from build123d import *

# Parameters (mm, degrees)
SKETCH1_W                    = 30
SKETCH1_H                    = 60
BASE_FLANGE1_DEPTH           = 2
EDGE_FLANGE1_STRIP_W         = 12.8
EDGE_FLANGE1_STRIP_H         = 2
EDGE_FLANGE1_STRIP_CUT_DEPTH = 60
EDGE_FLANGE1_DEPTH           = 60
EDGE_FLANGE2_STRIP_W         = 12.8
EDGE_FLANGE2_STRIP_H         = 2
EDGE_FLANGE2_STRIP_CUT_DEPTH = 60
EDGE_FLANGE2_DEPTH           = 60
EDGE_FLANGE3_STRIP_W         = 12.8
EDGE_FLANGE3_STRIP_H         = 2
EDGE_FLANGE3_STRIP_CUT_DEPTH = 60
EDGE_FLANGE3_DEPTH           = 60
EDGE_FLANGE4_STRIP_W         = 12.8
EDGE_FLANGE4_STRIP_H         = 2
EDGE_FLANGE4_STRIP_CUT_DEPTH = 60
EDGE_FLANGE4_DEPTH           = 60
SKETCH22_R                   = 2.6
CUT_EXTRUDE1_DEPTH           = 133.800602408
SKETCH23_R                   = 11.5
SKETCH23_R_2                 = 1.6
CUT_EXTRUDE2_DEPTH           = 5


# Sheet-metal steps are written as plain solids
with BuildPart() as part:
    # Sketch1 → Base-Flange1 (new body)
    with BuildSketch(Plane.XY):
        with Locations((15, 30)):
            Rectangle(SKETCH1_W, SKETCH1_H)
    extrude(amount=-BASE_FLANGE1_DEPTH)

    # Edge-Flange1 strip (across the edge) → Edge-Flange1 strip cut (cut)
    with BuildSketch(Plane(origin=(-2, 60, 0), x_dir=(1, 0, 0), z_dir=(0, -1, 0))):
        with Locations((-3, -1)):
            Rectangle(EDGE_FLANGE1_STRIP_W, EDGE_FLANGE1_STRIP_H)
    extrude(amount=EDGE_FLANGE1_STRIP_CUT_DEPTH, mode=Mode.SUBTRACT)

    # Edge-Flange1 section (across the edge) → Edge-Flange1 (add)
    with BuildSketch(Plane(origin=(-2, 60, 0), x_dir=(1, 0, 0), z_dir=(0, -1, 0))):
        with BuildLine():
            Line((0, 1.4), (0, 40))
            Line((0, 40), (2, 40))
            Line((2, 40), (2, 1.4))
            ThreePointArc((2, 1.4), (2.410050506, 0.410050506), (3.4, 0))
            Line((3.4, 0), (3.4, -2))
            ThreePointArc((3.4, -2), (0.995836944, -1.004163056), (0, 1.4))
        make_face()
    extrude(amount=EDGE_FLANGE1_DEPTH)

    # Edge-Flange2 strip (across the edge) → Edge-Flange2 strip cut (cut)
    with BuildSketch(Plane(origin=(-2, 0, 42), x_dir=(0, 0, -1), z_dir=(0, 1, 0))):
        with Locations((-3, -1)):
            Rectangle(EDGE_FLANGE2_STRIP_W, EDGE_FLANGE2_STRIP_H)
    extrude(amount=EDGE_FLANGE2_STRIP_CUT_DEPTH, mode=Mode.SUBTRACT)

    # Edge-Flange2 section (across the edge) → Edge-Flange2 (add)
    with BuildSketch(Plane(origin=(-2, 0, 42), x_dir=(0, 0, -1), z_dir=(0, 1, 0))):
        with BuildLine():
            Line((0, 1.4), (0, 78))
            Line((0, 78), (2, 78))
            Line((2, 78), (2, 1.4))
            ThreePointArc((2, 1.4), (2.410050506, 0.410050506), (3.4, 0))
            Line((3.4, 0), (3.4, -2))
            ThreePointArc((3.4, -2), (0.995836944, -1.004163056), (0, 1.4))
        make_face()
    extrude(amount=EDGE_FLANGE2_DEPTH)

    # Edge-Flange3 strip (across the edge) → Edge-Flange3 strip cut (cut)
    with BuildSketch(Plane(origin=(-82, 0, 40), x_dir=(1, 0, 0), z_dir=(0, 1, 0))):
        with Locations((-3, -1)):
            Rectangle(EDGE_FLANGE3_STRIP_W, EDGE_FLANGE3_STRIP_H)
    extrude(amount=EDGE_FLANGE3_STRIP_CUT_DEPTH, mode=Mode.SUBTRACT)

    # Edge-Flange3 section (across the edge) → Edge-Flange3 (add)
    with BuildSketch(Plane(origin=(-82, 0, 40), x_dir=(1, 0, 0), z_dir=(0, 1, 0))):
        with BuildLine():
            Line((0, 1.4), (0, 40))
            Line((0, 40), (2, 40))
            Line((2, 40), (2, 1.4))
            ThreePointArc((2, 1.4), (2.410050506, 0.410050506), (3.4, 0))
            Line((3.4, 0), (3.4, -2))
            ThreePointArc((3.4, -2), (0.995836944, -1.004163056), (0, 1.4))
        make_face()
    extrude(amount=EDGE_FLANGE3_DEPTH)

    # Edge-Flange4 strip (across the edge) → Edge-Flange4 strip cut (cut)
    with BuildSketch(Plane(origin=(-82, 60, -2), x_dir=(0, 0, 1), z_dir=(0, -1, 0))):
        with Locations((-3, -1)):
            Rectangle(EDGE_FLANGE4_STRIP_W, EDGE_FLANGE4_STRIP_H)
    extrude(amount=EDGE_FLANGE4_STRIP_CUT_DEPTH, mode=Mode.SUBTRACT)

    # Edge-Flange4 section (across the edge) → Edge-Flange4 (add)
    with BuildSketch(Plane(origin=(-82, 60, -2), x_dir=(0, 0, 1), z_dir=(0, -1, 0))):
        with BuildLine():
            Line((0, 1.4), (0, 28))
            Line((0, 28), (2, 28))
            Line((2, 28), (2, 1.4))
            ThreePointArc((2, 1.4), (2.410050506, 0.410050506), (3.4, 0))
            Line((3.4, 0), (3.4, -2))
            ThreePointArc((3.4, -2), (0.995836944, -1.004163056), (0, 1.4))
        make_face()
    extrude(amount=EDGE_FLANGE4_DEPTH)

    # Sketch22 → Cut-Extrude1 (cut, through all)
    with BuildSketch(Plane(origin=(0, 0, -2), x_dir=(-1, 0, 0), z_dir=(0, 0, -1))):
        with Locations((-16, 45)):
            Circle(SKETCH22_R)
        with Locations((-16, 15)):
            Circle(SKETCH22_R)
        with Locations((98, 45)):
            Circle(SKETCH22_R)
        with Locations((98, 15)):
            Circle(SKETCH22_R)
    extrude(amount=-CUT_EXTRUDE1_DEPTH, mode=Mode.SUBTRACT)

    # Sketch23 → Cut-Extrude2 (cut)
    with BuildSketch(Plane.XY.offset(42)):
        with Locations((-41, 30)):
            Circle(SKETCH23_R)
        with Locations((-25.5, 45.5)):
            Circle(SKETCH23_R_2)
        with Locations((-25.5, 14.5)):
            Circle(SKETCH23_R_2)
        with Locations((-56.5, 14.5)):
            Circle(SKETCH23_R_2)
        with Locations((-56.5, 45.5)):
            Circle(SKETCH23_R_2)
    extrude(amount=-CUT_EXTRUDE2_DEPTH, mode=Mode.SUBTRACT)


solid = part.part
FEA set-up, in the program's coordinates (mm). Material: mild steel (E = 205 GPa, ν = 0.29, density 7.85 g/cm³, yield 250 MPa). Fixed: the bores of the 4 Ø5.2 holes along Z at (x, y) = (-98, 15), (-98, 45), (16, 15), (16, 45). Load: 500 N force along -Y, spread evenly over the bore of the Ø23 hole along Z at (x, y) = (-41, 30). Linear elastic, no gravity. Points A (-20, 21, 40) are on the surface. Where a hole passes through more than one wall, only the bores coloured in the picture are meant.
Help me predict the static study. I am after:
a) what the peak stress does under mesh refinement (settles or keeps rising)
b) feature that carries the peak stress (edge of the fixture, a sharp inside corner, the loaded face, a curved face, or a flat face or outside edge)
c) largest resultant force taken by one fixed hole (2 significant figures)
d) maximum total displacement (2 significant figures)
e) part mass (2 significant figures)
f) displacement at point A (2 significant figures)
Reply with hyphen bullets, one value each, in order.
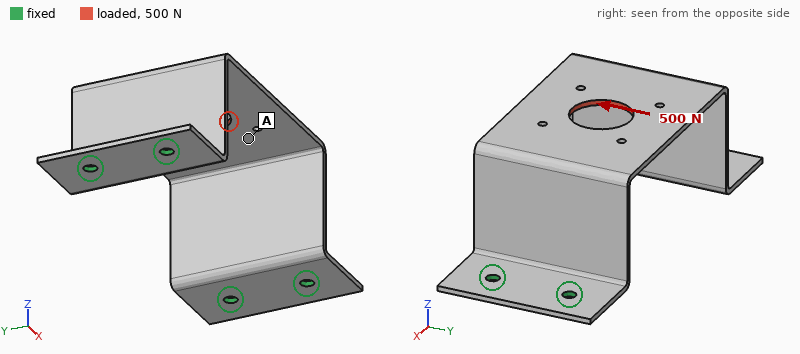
- keeps rising
- edge of the fixture
- 350 N
- 0.16 mm
- 200 g
- 0.13 mm
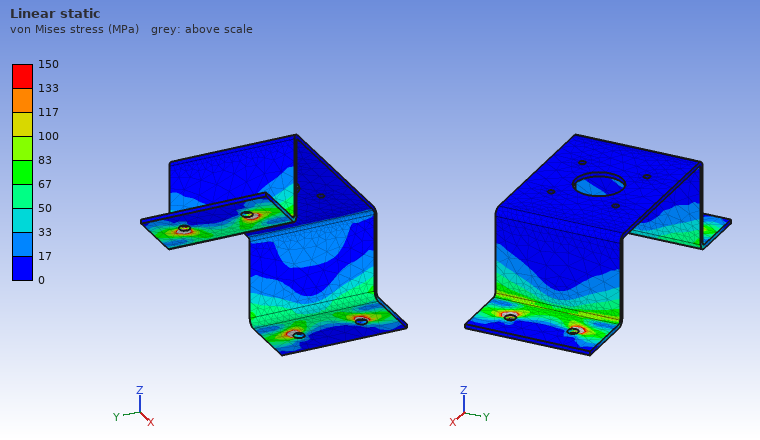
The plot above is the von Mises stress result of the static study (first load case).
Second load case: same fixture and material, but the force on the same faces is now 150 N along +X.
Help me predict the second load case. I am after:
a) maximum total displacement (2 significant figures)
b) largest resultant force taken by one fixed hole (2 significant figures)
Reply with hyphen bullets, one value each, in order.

- 0.14 mm
- 43 N
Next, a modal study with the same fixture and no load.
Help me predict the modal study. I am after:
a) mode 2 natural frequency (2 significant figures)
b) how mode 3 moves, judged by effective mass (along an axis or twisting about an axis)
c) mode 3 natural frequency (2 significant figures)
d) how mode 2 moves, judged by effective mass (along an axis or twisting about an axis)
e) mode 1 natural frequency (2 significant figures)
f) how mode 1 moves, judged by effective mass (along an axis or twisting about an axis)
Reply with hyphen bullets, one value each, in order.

- 900 Hz
- twisting about Z
- 1000 Hz
- along Y
- 530 Hz
- along X
